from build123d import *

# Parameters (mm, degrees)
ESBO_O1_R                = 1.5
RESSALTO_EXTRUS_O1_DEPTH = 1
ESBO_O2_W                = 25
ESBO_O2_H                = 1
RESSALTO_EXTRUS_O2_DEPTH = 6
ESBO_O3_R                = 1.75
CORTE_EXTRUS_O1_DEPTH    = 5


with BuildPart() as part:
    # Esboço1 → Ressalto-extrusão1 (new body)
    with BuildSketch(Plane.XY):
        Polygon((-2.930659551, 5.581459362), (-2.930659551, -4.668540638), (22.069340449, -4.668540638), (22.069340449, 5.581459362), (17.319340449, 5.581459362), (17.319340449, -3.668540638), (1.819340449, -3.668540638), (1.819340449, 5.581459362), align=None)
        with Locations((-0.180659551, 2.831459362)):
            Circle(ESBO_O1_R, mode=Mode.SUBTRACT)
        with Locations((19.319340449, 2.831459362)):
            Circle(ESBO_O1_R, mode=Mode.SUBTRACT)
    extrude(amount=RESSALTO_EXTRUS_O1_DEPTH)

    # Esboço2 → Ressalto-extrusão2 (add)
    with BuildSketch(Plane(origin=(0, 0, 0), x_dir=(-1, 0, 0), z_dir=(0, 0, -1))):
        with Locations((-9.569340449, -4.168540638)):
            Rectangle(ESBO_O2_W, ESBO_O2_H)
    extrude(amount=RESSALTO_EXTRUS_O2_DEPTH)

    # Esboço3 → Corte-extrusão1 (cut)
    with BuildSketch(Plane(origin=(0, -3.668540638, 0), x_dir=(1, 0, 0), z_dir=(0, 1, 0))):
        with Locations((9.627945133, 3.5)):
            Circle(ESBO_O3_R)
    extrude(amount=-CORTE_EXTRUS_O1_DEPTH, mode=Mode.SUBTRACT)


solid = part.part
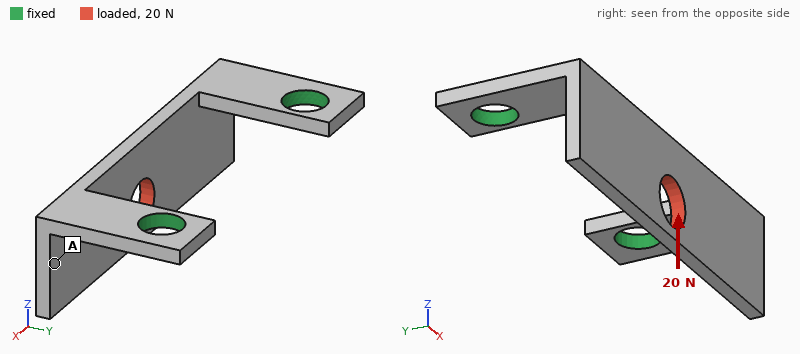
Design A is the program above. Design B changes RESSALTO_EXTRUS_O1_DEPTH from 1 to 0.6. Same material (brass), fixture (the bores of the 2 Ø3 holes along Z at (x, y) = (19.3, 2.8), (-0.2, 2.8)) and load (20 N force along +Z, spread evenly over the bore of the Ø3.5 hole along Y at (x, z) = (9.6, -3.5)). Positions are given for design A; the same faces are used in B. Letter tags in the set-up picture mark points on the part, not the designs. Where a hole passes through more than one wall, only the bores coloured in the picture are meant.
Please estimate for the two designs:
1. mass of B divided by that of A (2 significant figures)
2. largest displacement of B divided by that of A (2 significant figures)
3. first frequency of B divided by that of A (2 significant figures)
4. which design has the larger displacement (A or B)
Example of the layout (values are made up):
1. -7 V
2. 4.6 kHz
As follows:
1. 0.83
2. 4.2
3. 0.51
4. B
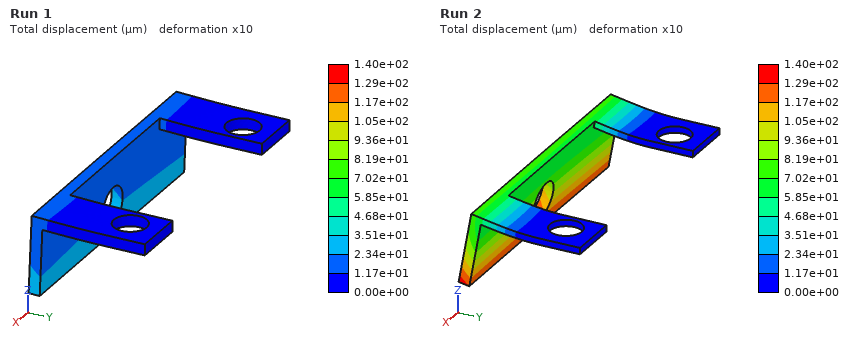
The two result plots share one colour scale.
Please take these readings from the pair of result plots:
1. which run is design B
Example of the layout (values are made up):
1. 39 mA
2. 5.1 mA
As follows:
1. Run 2
